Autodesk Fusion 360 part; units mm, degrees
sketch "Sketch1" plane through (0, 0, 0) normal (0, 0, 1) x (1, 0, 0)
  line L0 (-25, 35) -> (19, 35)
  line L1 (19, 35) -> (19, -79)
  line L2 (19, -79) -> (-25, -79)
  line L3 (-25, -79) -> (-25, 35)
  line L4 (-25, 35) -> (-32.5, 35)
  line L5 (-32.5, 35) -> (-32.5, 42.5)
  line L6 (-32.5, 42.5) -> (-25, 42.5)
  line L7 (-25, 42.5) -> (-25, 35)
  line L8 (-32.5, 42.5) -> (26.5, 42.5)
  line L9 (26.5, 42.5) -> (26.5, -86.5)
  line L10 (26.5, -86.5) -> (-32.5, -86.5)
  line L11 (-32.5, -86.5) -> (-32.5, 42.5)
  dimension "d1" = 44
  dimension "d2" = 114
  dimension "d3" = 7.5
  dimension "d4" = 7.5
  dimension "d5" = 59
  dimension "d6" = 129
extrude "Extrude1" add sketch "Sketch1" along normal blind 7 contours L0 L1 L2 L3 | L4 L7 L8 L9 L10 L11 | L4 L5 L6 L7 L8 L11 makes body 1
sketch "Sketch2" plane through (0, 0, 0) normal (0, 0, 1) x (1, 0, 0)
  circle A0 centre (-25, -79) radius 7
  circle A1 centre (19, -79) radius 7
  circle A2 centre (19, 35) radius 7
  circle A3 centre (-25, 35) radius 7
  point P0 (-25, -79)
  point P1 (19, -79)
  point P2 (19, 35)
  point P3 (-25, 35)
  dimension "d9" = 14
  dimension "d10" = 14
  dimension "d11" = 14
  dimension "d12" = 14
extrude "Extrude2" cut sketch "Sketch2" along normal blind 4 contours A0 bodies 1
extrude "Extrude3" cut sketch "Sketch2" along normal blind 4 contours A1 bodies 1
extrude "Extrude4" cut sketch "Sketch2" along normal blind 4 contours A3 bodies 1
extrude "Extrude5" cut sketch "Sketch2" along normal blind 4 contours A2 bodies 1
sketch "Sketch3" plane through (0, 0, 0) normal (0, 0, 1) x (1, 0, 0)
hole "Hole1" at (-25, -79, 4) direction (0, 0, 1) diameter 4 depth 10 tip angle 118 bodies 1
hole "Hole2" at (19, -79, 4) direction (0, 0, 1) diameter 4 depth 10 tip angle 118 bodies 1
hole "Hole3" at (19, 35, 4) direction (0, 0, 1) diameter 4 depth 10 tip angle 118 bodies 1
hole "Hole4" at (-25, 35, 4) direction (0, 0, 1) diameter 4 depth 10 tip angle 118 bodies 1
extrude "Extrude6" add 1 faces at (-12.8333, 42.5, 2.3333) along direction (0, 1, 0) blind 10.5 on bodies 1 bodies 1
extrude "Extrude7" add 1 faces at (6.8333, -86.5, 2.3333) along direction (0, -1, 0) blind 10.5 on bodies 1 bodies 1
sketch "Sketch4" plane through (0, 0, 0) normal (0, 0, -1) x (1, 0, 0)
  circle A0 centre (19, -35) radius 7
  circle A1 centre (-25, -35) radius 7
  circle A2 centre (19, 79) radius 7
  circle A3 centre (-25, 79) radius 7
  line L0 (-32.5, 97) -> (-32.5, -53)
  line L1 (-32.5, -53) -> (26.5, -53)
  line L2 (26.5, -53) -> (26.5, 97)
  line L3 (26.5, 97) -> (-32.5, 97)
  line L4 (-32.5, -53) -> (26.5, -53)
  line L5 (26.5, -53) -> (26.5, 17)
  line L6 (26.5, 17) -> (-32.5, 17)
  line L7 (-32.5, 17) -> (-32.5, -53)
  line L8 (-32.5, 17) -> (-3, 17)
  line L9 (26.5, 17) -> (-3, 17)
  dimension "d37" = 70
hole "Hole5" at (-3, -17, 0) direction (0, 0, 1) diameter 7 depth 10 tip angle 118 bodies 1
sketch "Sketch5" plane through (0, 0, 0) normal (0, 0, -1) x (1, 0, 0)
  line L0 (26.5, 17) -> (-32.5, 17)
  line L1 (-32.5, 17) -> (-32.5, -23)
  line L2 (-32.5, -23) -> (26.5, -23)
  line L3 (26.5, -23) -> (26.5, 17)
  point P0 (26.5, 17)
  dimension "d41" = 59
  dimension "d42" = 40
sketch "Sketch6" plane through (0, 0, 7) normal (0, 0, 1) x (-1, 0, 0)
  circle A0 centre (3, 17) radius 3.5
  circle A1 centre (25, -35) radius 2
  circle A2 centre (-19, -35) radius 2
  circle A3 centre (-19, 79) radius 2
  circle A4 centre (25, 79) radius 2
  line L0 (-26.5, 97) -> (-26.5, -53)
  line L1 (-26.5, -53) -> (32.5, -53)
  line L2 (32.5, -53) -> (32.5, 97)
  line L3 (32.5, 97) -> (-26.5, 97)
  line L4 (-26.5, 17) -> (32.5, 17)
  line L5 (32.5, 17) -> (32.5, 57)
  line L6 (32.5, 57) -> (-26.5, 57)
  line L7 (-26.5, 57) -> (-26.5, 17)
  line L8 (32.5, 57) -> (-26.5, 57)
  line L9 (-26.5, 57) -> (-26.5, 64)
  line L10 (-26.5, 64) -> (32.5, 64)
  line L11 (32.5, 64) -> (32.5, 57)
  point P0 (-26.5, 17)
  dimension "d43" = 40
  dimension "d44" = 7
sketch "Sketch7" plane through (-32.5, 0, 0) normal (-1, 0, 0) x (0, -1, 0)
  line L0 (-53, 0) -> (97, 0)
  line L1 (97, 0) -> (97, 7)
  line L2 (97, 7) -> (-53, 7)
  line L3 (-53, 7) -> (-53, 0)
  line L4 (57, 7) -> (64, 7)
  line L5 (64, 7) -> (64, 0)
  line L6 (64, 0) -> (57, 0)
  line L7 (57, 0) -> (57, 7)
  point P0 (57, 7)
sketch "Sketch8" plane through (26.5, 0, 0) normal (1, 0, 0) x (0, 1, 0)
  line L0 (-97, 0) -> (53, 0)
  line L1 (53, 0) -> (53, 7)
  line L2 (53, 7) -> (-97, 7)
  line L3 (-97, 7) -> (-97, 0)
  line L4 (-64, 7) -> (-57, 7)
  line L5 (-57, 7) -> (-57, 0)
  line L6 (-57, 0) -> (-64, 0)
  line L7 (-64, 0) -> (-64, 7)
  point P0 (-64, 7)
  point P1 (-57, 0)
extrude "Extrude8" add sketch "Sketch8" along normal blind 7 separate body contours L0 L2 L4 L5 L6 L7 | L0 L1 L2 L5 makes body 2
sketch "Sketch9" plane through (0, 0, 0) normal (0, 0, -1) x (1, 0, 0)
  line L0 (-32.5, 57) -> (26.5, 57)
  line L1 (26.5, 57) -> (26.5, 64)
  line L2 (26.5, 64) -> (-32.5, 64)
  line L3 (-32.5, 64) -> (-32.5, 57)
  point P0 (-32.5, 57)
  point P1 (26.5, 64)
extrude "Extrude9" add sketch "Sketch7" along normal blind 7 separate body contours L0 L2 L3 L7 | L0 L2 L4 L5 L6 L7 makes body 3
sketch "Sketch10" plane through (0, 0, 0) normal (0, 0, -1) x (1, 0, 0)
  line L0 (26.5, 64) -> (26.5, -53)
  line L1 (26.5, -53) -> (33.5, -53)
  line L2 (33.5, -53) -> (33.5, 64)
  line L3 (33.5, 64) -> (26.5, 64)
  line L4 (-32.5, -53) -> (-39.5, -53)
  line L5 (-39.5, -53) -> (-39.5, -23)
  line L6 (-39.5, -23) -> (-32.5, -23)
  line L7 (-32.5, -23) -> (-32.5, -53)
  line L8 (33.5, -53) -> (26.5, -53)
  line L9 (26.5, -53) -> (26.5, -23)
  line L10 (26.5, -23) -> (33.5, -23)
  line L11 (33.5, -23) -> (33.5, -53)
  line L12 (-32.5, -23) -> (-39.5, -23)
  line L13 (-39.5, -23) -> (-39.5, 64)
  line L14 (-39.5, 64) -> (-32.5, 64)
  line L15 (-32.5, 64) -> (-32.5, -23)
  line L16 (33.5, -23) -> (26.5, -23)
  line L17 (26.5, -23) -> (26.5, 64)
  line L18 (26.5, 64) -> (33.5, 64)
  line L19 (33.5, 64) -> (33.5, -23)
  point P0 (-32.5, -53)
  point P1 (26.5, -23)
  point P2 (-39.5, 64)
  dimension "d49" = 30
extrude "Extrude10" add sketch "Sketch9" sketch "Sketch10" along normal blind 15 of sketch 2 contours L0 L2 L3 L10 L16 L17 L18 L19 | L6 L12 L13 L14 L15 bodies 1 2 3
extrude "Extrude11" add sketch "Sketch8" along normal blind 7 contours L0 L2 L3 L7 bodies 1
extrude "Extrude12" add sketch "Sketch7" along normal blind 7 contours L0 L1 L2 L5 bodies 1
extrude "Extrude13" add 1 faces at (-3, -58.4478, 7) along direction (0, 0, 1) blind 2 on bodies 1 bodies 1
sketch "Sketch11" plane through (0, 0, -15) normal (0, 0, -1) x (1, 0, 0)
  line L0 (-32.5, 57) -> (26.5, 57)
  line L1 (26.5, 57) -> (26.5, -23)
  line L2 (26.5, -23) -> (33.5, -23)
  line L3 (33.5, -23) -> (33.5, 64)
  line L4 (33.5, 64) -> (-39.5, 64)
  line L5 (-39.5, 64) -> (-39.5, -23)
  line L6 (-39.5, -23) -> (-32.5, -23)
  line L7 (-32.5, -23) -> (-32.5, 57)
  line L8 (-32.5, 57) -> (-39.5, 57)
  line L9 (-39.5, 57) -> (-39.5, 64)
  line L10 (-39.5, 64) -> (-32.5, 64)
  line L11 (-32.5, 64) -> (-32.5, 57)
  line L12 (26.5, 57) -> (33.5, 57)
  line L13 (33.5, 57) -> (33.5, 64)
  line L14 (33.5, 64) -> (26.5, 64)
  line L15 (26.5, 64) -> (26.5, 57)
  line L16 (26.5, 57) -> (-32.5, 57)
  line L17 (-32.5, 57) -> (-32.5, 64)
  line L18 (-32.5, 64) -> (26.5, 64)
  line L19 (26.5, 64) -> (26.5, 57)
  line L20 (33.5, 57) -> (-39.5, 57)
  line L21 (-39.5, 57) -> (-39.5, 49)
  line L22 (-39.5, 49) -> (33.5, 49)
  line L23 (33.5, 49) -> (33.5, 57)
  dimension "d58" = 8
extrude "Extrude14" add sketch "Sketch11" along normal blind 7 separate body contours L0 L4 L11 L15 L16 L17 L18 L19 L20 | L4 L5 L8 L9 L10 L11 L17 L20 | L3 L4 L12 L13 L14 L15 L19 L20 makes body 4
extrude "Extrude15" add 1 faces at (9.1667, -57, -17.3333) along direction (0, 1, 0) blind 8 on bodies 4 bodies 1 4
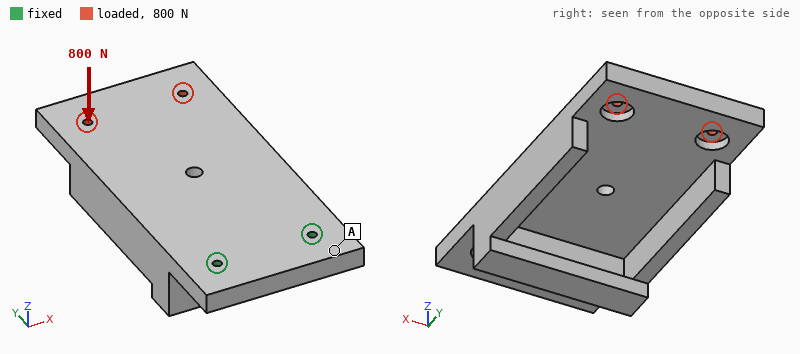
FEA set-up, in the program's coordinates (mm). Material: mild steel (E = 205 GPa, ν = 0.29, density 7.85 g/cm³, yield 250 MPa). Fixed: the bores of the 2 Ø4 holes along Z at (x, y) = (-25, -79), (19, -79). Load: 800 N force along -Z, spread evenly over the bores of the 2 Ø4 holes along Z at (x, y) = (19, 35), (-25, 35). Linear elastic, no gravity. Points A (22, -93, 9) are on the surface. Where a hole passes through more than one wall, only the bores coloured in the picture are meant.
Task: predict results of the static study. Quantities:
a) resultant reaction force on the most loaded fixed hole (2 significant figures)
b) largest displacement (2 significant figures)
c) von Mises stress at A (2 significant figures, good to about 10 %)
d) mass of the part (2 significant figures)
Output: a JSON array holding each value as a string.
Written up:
["520 N", "0.67 mm", "32 MPa", "1.0 kg"]
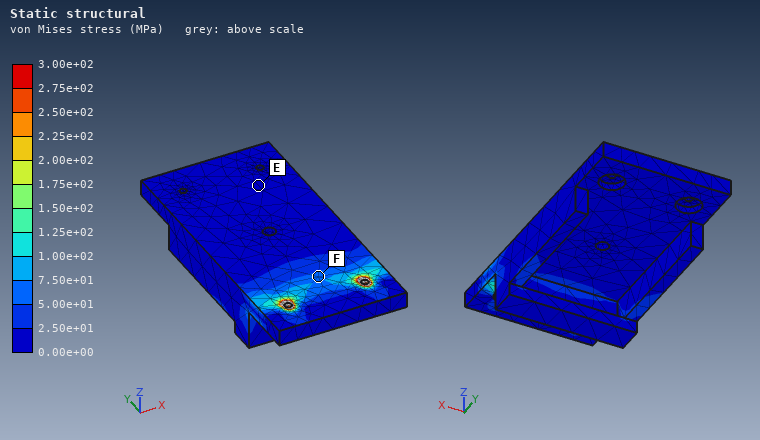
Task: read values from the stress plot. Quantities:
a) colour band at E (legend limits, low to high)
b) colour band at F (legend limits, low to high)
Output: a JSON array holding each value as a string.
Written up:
["0.00e+00 to 2.50e+01 MPa", "5.00e+01 to 7.50e+01 MPa"]
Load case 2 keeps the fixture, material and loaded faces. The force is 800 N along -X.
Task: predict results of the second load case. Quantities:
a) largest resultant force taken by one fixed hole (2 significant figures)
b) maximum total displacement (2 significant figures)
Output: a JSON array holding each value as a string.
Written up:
["2.1 kN", "17 µm"]
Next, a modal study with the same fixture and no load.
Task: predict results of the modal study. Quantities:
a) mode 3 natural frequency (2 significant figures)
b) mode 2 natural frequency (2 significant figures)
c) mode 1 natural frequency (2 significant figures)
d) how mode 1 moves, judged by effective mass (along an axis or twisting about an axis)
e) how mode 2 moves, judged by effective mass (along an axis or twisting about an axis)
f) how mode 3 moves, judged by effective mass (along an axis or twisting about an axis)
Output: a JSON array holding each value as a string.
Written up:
["2100 Hz", "1600 Hz", "330 Hz", "along Z", "twisting about Y", "along X"]
